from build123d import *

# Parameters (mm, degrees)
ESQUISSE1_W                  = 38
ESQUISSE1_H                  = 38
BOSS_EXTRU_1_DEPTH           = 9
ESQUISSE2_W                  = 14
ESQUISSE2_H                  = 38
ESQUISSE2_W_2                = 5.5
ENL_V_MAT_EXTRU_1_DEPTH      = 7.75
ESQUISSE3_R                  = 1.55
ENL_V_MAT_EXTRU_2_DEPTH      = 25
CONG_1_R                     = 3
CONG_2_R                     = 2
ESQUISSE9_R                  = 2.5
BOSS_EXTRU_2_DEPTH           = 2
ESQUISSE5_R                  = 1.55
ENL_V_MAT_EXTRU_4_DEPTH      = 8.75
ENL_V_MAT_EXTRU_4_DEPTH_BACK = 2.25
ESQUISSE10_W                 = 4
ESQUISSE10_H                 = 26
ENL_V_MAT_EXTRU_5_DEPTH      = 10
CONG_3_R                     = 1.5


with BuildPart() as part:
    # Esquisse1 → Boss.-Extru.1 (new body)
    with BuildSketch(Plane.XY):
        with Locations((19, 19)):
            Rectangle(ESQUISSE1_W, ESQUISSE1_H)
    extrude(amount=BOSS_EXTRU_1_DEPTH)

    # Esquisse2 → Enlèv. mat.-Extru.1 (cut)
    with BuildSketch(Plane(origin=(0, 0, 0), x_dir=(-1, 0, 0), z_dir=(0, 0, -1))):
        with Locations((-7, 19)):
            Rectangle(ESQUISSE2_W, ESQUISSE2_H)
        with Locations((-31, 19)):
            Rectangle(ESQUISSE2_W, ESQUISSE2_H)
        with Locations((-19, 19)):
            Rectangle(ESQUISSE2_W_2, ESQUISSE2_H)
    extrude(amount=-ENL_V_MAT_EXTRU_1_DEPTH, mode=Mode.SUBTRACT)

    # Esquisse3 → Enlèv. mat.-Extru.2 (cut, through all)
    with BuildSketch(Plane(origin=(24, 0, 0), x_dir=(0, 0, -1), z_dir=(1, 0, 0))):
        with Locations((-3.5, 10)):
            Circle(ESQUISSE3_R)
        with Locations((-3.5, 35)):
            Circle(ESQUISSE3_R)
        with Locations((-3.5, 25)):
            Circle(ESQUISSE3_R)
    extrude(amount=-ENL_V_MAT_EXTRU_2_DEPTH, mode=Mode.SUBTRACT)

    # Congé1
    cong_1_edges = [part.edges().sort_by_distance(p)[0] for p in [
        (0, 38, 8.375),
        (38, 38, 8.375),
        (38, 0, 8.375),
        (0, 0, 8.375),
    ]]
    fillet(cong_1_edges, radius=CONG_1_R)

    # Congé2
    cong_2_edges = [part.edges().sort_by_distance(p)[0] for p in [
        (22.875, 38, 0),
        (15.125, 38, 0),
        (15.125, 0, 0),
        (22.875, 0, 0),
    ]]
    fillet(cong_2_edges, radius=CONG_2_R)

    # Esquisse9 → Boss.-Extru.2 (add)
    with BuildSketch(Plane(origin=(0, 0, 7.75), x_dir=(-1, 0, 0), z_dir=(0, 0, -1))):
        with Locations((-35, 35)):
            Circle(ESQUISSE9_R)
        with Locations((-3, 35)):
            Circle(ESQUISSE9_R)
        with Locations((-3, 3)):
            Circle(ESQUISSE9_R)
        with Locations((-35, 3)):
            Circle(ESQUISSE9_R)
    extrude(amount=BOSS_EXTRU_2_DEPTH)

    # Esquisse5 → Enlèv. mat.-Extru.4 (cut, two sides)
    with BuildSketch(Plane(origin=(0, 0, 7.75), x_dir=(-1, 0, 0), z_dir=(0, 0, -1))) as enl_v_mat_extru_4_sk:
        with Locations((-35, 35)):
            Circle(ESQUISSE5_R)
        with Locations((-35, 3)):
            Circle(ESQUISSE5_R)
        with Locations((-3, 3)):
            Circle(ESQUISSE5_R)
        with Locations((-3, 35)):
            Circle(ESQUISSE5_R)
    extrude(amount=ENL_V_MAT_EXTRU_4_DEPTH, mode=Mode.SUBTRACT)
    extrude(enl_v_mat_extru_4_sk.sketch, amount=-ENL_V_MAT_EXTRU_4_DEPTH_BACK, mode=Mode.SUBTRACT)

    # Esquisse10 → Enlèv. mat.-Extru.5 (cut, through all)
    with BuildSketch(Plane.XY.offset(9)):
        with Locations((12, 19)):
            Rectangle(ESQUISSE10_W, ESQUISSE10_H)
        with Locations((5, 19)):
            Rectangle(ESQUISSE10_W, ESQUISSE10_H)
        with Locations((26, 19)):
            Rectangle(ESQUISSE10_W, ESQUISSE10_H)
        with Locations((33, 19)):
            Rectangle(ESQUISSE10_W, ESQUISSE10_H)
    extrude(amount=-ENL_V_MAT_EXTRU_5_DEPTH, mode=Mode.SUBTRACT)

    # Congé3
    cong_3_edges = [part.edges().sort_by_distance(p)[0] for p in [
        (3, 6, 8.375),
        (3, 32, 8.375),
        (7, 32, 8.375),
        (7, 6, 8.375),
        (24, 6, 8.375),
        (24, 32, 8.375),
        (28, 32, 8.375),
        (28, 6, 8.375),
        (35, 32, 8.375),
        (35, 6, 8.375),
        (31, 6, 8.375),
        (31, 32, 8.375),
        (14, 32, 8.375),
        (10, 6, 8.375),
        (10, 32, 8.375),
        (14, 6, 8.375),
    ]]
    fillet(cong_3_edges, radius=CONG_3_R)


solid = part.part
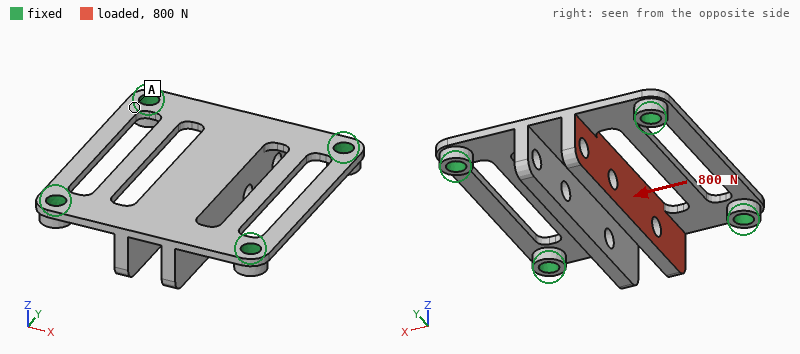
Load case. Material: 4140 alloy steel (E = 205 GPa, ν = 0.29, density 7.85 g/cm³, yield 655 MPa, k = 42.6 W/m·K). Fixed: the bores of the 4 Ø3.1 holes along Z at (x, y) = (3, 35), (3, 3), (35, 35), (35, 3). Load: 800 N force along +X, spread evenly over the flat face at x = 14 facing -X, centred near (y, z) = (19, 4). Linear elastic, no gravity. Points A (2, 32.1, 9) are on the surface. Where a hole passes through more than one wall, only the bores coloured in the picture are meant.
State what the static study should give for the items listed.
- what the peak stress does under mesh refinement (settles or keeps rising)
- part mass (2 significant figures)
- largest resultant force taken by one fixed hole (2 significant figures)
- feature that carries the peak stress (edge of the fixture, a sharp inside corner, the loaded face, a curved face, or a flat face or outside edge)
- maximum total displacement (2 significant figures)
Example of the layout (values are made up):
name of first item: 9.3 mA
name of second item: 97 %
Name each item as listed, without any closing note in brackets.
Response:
what the peak stress does under mesh refinement: keeps rising
part mass: 20 g
largest resultant force taken by one fixed hole: 240 N
feature that carries the peak stress: a sharp inside corner
maximum total displacement: 79 µm
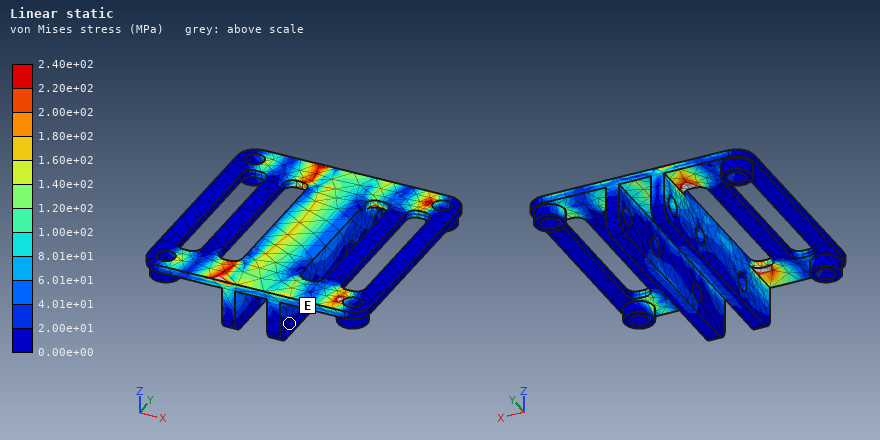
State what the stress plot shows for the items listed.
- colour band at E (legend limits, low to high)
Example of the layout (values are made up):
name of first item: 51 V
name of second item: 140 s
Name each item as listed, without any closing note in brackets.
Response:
colour band at E: 0.00e+00 to 2.00e+01 MPa
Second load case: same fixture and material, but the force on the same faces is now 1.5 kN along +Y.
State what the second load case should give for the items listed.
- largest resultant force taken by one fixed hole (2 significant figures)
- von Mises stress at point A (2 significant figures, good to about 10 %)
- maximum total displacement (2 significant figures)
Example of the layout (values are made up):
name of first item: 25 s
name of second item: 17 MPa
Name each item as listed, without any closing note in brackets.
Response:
largest resultant force taken by one fixed hole: 420 N
von Mises stress at point A: 36 MPa
maximum total displacement: 77 µm
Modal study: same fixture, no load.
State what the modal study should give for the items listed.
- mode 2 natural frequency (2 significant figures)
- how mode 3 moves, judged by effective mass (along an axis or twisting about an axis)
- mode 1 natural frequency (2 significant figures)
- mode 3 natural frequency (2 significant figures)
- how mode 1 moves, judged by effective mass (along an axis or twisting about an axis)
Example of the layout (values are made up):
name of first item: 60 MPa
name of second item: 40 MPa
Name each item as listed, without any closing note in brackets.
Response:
mode 2 natural frequency: 5100 Hz
how mode 3 moves, judged by effective mass: along X
mode 1 natural frequency: 3500 Hz
mode 3 natural frequency: 6500 Hz
how mode 1 moves, judged by effective mass: along Z
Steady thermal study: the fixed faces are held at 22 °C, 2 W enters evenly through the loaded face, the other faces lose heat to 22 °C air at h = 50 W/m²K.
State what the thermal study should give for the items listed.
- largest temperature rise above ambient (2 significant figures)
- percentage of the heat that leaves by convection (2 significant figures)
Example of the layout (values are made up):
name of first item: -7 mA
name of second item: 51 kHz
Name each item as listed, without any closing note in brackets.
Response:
largest temperature rise above ambient: 14 K
percentage of the heat that leaves by convection: 51 %
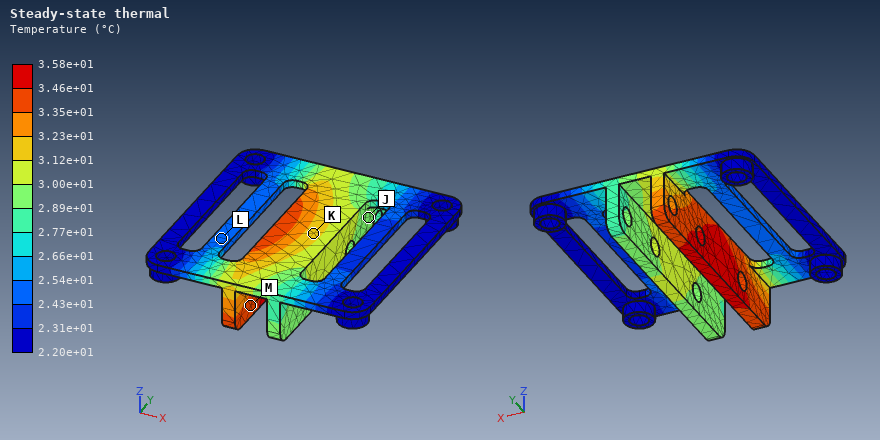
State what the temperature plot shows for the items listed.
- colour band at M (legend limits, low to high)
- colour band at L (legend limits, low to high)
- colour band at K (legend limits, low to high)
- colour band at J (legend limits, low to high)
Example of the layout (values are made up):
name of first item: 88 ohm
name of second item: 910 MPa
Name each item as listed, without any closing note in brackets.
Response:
colour band at M: 3.35e+01 to 3.46e+01 °C
colour band at L: 2.43e+01 to 2.54e+01 °C
colour band at K: 3.12e+01 to 3.23e+01 °C
colour band at J: 2.89e+01 to 3.00e+01 °C
